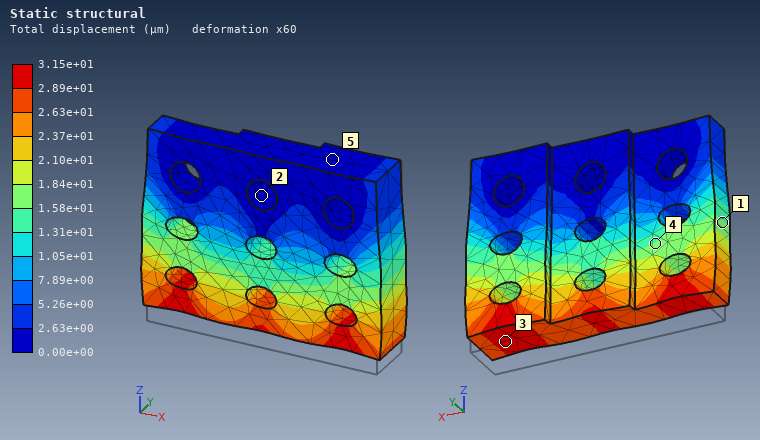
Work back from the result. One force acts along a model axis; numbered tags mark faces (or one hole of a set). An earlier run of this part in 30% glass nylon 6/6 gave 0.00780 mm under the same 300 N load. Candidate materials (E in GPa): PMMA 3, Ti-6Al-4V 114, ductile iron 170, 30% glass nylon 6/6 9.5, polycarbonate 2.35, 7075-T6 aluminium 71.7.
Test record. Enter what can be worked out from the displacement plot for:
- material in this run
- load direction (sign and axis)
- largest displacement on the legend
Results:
polycarbonate
+Z
3.15e+01 µm
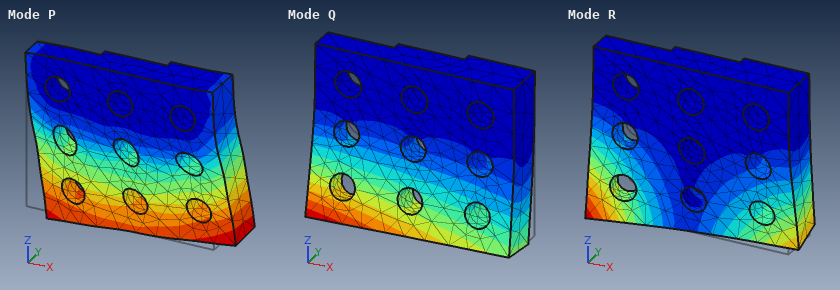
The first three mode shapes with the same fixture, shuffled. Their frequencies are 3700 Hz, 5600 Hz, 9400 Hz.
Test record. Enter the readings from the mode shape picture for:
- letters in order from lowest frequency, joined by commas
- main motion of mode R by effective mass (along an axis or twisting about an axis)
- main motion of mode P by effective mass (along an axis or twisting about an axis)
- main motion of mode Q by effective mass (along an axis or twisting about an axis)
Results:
Q, R, P
twisting about Z
along X
along Y
